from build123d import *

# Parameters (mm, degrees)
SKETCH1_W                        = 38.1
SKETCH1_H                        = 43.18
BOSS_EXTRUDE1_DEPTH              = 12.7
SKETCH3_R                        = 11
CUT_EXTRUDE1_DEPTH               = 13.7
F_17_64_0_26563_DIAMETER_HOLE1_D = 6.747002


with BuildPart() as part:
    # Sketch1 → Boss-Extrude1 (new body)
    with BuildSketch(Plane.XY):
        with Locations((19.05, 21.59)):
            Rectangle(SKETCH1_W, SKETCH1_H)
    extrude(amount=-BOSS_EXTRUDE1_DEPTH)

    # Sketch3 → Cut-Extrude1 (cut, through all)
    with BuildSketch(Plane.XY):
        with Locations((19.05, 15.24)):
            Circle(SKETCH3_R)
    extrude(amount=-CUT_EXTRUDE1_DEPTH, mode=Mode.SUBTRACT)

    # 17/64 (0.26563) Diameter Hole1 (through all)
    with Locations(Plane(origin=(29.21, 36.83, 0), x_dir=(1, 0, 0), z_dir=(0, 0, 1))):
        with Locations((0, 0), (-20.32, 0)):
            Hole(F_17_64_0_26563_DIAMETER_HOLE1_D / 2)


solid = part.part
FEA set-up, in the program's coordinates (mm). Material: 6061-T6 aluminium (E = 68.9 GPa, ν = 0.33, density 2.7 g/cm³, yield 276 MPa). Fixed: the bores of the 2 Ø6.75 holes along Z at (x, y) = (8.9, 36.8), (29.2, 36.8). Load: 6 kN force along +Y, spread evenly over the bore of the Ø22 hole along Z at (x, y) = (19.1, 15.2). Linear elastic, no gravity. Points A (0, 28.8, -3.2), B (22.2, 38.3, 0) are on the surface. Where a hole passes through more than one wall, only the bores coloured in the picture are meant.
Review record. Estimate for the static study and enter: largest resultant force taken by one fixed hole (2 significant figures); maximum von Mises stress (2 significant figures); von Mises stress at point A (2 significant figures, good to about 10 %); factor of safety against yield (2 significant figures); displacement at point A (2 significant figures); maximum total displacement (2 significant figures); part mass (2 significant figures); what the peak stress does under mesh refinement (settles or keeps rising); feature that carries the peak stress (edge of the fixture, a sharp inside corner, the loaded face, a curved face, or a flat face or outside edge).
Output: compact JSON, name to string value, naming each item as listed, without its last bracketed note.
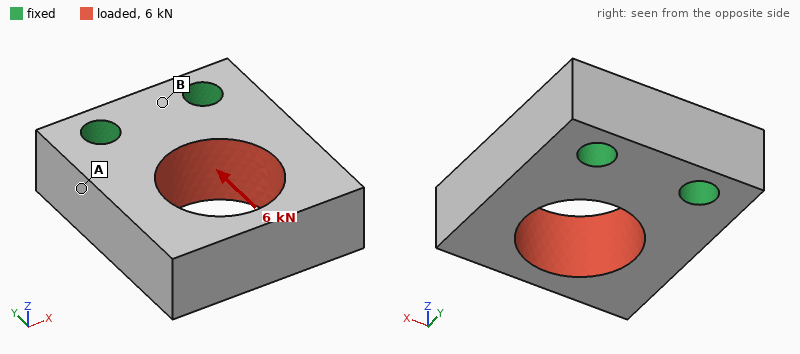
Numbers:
{"largest resultant force taken by one fixed hole": "3.0 kN", "maximum von Mises stress": "52 MPa", "von Mises stress at point A": "18 MPa", "factor of safety against yield": "5.3", "displacement at point A": "4.5 µm", "maximum total displacement": "21 µm", "part mass": "41 g", "what the peak stress does under mesh refinement": "settles", "feature that carries the peak stress": "the loaded face"}
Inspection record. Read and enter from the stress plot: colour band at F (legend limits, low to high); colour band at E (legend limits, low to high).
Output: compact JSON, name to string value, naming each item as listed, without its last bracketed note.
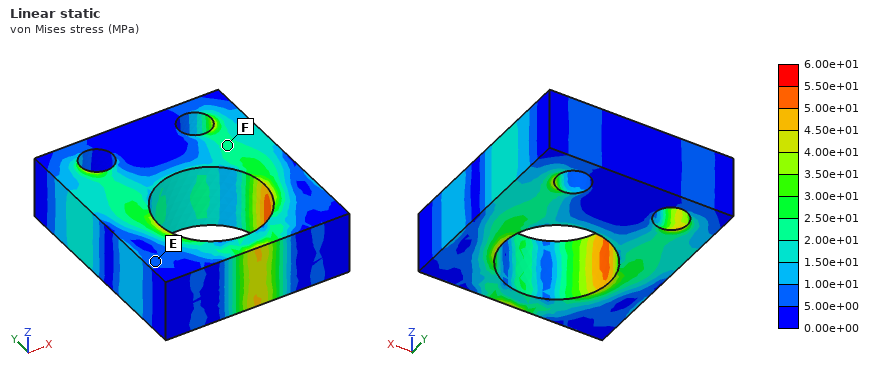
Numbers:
{"colour band at F": "2.00e+01 to 2.50e+01 MPa", "colour band at E": "5.00e+00 to 1.00e+01 MPa"}
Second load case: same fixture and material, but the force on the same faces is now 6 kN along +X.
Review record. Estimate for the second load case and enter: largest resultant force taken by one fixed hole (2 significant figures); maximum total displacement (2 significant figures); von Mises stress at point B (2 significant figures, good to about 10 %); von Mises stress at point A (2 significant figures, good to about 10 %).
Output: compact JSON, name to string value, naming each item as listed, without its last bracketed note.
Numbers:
{"largest resultant force taken by one fixed hole": "5.0 kN", "maximum total displacement": "82 µm", "von Mises stress at point B": "10 MPa", "von Mises stress at point A": "62 MPa"}
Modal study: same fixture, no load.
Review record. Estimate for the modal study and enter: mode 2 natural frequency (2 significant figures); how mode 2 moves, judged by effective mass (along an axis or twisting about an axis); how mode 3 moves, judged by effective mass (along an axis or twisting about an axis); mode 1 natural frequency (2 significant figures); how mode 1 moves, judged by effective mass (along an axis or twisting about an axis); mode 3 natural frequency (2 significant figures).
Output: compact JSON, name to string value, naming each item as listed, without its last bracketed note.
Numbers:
{"mode 2 natural frequency": "9500 Hz", "how mode 2 moves, judged by effective mass": "along X", "how mode 3 moves, judged by effective mass": "twisting about Y", "mode 1 natural frequency": "7000 Hz", "how mode 1 moves, judged by effective mass": "along Z", "mode 3 natural frequency": "11 kHz"}
